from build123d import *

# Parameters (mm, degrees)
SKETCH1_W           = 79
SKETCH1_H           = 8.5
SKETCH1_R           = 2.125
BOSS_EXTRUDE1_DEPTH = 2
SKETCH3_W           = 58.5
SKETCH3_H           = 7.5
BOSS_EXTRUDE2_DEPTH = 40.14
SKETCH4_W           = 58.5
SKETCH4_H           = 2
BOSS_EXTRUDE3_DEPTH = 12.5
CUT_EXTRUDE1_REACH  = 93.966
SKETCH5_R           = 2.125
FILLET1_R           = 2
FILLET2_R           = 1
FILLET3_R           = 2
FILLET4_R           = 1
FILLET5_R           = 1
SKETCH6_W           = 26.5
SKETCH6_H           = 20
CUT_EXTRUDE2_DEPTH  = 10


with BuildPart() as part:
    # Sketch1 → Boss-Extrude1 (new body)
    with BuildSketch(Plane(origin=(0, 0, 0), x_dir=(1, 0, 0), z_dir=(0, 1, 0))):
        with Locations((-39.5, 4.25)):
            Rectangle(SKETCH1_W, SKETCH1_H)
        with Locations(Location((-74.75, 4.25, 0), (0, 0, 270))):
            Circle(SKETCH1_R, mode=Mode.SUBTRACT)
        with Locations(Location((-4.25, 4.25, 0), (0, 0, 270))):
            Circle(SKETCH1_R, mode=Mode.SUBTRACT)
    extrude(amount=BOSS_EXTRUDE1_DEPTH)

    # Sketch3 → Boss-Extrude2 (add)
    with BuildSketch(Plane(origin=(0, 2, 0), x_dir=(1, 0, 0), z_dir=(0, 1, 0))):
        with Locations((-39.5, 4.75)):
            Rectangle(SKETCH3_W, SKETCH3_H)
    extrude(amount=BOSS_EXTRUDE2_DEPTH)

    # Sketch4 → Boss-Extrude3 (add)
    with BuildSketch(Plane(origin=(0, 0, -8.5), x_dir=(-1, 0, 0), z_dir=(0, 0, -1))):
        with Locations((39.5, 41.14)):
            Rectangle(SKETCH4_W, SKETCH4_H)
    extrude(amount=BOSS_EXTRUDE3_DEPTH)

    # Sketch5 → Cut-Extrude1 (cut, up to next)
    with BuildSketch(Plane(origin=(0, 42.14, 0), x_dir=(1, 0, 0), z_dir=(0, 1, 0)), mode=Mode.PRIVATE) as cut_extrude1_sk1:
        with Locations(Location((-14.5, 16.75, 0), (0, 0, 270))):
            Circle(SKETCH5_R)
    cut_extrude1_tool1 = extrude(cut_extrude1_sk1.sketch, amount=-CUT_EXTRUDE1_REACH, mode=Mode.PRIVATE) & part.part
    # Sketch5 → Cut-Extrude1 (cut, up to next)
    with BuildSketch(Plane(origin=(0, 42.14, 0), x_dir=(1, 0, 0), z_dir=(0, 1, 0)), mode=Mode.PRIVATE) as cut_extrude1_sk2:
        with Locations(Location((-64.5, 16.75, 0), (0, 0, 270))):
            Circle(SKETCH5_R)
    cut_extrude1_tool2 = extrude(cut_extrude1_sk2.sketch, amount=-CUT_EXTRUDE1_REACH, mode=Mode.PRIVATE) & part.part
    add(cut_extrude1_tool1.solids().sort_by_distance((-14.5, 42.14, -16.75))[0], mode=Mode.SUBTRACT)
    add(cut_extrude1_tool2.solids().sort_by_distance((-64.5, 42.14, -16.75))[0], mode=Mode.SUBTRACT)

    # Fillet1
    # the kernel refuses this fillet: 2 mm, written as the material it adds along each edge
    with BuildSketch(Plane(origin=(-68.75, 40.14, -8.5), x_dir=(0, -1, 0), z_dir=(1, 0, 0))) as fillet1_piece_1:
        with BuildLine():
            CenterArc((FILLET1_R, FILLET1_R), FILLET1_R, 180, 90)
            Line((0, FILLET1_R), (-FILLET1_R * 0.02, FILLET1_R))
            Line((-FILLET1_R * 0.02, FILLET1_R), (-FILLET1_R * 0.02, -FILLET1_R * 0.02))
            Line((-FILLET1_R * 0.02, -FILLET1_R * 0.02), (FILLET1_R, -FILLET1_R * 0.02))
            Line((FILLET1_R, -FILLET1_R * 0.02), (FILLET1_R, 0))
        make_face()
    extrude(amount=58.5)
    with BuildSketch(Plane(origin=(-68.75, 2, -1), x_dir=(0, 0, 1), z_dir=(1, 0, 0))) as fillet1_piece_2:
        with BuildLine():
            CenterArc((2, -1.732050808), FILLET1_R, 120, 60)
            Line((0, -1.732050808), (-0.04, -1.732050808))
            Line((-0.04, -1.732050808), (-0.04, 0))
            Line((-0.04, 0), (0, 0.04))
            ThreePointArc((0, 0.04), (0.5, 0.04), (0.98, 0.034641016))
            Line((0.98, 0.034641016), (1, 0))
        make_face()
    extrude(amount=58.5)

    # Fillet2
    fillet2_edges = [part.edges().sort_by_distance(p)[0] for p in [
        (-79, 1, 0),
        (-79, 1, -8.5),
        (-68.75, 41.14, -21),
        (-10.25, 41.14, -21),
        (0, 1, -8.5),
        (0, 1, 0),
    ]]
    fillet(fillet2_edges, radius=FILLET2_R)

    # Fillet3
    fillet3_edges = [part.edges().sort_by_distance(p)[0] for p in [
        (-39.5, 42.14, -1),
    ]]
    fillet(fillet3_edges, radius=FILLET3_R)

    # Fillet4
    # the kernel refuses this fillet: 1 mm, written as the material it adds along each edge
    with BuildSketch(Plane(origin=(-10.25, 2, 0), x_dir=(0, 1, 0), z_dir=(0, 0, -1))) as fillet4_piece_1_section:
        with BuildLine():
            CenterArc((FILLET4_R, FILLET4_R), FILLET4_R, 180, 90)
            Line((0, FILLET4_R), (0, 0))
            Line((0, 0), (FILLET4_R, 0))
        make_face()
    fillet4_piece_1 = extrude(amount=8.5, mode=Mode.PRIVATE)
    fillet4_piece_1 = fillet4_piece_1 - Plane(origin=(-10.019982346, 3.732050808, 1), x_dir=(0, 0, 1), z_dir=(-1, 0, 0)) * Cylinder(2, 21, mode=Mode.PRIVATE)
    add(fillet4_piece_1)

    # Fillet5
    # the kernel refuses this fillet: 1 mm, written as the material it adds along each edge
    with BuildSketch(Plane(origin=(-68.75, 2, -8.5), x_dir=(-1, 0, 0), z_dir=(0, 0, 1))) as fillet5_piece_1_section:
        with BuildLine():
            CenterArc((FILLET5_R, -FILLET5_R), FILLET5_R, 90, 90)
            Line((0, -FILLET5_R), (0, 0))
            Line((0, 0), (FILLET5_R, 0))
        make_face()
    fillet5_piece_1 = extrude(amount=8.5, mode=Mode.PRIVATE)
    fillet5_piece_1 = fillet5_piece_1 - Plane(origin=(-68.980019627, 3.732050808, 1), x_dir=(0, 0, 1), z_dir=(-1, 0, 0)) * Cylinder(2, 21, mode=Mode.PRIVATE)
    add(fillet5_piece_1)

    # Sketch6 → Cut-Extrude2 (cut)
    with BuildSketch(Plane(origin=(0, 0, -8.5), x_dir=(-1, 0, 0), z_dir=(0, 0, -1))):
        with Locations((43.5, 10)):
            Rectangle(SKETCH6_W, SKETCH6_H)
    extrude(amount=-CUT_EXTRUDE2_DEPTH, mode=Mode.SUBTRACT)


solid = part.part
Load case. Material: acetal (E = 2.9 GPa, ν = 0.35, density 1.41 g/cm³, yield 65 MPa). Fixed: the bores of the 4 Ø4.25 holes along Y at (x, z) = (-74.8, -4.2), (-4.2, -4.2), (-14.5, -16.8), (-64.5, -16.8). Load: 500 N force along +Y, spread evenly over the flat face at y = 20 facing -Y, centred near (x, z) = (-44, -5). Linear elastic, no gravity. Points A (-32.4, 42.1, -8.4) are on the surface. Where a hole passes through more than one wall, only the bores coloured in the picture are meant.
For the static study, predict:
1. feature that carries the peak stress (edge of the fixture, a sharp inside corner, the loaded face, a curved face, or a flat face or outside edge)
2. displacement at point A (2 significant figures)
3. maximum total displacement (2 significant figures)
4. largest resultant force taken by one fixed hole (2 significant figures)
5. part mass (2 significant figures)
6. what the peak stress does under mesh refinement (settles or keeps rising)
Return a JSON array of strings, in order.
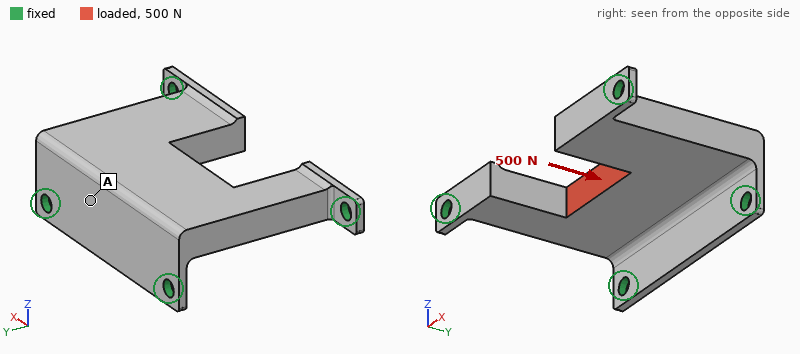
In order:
["edge of the fixture", "0.19 mm", "0.25 mm", "200 N", "23 g", "keeps rising"]
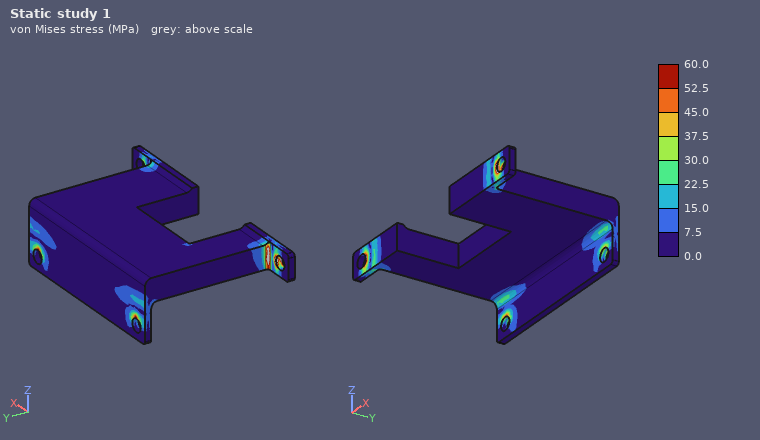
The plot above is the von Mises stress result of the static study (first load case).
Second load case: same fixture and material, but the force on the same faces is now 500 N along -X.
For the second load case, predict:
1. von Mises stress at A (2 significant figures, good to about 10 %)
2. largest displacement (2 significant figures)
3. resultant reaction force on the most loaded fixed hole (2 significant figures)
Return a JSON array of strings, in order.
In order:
["3.0 MPa", "0.12 mm", "170 N"]
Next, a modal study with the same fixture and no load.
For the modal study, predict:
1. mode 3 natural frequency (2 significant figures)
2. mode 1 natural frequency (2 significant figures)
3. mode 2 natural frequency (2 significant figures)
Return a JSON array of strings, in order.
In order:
["2700 Hz", "1600 Hz", "1900 Hz"]
